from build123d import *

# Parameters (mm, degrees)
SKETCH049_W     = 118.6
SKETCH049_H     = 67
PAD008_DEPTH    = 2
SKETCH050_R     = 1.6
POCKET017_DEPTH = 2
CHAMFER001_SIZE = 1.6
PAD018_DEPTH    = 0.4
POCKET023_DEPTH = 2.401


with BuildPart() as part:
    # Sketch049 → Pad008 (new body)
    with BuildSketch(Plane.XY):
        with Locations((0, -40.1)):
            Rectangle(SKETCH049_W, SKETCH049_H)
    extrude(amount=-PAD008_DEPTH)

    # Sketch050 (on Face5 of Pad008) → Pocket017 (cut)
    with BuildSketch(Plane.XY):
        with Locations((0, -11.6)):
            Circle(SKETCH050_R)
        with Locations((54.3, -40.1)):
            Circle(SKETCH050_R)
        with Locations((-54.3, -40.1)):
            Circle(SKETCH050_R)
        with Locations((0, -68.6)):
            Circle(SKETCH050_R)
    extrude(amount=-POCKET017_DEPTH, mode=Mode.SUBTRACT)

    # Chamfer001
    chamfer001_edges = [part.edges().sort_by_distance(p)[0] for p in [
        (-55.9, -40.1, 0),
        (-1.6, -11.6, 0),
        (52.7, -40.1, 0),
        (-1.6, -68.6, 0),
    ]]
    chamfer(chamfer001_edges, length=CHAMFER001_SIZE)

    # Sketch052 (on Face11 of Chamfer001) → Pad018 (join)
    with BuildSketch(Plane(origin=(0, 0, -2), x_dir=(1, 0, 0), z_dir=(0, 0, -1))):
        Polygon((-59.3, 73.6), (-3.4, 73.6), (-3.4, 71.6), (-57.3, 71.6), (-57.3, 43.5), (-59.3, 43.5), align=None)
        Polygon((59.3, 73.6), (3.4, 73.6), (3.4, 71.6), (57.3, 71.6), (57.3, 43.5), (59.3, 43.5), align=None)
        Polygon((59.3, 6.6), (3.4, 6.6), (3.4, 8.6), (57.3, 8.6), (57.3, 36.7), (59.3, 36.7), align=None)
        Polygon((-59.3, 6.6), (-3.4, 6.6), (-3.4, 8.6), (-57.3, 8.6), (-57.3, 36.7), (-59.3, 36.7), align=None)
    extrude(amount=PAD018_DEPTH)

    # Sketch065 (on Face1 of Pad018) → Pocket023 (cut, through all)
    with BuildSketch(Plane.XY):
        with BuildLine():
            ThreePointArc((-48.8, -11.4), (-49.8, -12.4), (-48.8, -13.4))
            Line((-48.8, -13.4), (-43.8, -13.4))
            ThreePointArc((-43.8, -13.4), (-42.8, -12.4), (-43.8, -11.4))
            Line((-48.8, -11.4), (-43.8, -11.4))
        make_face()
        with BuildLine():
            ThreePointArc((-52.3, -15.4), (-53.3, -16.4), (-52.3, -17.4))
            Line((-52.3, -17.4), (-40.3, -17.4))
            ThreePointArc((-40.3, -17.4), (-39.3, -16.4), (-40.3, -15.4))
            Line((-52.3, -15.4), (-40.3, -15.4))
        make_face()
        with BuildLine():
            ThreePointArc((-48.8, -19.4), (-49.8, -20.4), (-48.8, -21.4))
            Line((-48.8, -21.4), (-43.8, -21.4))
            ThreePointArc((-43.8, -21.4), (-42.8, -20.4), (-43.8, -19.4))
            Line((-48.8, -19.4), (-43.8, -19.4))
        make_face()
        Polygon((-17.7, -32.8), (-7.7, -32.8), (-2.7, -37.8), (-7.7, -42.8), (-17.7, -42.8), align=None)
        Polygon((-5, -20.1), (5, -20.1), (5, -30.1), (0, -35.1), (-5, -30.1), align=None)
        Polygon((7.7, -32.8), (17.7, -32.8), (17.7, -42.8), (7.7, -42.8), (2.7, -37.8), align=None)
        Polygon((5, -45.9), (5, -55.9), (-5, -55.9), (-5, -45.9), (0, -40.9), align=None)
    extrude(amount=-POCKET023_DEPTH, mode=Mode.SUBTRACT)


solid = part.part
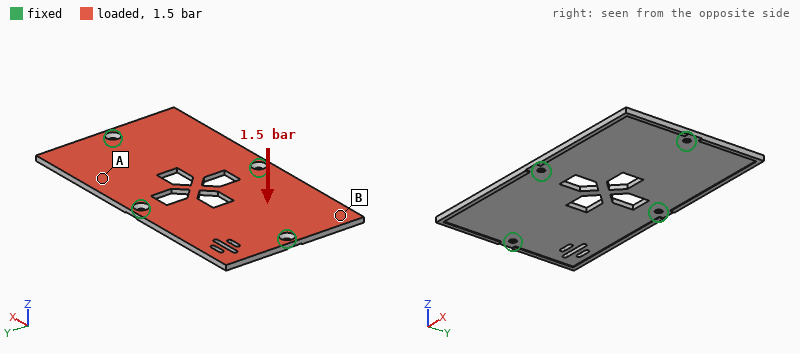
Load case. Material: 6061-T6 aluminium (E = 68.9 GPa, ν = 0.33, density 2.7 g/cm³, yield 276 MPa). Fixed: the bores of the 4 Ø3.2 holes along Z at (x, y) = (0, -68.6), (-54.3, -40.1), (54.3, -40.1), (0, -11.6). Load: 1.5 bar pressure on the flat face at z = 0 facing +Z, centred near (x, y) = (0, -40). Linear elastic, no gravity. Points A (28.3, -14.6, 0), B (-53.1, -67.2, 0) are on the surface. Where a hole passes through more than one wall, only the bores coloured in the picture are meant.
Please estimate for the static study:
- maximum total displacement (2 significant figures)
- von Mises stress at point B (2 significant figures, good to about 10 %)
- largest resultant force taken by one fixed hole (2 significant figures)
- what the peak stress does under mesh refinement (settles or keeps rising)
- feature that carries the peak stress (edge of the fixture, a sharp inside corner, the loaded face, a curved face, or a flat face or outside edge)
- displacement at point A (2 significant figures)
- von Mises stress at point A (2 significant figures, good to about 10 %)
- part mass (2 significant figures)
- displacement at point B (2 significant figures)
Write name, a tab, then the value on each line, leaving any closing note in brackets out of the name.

maximum total displacement	0.37 mm
von Mises stress at point B	22 MPa
largest resultant force taken by one fixed hole	570 N
what the peak stress does under mesh refinement	keeps rising
feature that carries the peak stress	edge of the fixture
displacement at point A	0.25 mm
von Mises stress at point A	54 MPa
part mass	40 g
displacement at point B	0.28 mm
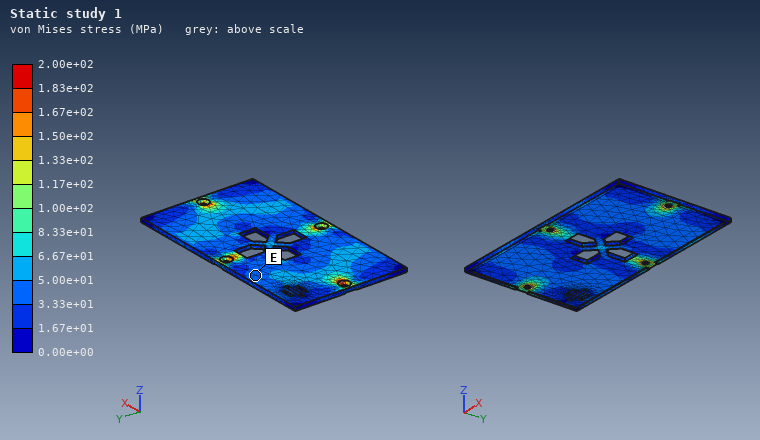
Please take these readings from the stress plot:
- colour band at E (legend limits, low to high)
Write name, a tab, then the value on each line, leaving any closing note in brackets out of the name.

colour band at E	3.33e+01 to 5.00e+01 MPa
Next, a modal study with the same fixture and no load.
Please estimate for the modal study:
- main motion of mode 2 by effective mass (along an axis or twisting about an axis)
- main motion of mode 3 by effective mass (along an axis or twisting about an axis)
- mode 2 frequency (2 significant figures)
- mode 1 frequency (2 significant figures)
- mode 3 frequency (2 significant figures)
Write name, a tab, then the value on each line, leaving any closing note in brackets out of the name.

main motion of mode 2 by effective mass	twisting about X
main motion of mode 3 by effective mass	twisting about Y
mode 2 frequency	1300 Hz
mode 1 frequency	1300 Hz
mode 3 frequency	1600 Hz
